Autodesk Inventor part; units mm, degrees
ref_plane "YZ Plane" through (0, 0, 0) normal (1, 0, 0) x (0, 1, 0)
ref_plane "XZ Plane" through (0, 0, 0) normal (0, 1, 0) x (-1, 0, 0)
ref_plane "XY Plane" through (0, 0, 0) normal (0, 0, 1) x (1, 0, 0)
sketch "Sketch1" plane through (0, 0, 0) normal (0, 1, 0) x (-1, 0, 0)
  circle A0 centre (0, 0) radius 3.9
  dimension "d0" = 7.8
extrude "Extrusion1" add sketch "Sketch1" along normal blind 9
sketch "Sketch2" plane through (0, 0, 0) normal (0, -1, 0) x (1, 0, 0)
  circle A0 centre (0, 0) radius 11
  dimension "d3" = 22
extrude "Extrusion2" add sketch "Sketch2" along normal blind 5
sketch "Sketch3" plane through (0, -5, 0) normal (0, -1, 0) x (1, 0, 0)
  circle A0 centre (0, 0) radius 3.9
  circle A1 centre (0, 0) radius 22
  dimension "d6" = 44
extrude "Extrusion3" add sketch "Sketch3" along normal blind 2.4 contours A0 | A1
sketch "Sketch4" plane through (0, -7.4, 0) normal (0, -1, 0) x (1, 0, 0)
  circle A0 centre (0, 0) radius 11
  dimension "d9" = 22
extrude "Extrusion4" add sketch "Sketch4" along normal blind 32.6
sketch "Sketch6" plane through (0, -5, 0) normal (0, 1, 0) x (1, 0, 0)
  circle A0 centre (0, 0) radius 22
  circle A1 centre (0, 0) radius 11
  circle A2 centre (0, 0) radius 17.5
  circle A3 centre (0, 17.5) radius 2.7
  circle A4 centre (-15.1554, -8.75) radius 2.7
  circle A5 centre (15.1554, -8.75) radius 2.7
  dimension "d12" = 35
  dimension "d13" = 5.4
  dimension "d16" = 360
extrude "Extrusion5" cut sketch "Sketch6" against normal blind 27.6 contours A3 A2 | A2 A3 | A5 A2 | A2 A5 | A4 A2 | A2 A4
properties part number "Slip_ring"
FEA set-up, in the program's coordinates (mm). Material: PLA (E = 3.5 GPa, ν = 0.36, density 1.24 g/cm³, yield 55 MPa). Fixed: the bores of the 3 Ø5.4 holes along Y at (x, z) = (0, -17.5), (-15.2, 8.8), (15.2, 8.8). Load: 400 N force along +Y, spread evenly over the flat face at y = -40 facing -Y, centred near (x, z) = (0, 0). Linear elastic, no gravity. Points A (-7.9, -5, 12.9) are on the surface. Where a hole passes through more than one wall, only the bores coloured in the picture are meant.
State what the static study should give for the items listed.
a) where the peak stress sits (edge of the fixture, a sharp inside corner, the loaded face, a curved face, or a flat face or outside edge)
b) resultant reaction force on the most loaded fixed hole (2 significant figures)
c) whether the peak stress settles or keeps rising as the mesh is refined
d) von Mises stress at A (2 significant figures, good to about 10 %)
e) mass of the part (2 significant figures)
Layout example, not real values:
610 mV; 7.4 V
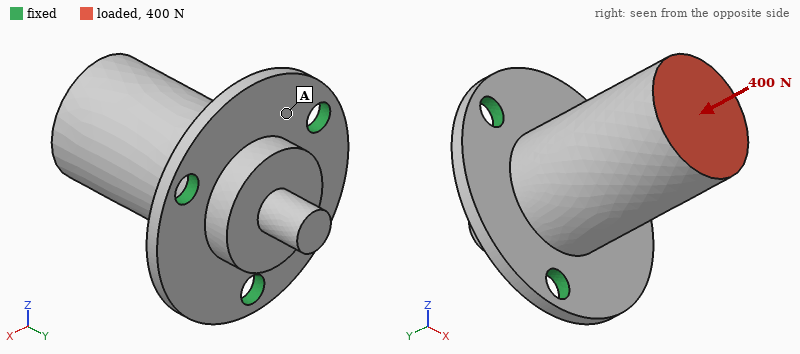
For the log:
edge of the fixture; 130 N; keeps rising; 3.5 MPa; 23 g
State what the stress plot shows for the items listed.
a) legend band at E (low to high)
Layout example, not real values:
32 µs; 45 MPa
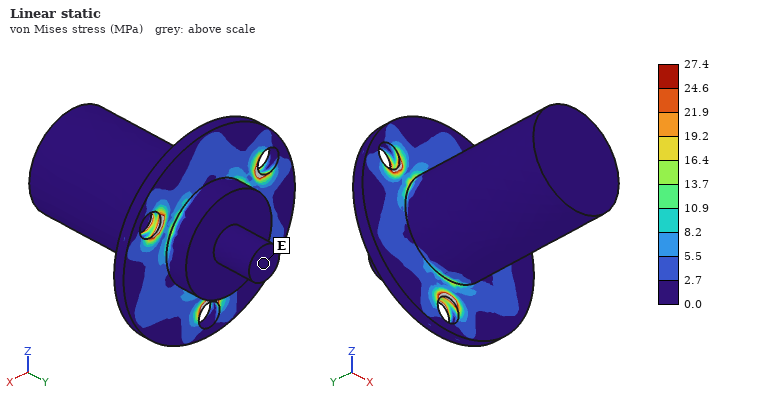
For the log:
0.0 to 2.7 MPa
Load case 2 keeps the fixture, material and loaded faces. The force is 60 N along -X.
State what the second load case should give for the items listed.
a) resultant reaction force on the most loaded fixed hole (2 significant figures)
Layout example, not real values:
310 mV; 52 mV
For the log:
83 N
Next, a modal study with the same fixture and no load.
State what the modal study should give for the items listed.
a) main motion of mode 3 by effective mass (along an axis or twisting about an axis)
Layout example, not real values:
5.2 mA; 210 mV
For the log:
along Y
